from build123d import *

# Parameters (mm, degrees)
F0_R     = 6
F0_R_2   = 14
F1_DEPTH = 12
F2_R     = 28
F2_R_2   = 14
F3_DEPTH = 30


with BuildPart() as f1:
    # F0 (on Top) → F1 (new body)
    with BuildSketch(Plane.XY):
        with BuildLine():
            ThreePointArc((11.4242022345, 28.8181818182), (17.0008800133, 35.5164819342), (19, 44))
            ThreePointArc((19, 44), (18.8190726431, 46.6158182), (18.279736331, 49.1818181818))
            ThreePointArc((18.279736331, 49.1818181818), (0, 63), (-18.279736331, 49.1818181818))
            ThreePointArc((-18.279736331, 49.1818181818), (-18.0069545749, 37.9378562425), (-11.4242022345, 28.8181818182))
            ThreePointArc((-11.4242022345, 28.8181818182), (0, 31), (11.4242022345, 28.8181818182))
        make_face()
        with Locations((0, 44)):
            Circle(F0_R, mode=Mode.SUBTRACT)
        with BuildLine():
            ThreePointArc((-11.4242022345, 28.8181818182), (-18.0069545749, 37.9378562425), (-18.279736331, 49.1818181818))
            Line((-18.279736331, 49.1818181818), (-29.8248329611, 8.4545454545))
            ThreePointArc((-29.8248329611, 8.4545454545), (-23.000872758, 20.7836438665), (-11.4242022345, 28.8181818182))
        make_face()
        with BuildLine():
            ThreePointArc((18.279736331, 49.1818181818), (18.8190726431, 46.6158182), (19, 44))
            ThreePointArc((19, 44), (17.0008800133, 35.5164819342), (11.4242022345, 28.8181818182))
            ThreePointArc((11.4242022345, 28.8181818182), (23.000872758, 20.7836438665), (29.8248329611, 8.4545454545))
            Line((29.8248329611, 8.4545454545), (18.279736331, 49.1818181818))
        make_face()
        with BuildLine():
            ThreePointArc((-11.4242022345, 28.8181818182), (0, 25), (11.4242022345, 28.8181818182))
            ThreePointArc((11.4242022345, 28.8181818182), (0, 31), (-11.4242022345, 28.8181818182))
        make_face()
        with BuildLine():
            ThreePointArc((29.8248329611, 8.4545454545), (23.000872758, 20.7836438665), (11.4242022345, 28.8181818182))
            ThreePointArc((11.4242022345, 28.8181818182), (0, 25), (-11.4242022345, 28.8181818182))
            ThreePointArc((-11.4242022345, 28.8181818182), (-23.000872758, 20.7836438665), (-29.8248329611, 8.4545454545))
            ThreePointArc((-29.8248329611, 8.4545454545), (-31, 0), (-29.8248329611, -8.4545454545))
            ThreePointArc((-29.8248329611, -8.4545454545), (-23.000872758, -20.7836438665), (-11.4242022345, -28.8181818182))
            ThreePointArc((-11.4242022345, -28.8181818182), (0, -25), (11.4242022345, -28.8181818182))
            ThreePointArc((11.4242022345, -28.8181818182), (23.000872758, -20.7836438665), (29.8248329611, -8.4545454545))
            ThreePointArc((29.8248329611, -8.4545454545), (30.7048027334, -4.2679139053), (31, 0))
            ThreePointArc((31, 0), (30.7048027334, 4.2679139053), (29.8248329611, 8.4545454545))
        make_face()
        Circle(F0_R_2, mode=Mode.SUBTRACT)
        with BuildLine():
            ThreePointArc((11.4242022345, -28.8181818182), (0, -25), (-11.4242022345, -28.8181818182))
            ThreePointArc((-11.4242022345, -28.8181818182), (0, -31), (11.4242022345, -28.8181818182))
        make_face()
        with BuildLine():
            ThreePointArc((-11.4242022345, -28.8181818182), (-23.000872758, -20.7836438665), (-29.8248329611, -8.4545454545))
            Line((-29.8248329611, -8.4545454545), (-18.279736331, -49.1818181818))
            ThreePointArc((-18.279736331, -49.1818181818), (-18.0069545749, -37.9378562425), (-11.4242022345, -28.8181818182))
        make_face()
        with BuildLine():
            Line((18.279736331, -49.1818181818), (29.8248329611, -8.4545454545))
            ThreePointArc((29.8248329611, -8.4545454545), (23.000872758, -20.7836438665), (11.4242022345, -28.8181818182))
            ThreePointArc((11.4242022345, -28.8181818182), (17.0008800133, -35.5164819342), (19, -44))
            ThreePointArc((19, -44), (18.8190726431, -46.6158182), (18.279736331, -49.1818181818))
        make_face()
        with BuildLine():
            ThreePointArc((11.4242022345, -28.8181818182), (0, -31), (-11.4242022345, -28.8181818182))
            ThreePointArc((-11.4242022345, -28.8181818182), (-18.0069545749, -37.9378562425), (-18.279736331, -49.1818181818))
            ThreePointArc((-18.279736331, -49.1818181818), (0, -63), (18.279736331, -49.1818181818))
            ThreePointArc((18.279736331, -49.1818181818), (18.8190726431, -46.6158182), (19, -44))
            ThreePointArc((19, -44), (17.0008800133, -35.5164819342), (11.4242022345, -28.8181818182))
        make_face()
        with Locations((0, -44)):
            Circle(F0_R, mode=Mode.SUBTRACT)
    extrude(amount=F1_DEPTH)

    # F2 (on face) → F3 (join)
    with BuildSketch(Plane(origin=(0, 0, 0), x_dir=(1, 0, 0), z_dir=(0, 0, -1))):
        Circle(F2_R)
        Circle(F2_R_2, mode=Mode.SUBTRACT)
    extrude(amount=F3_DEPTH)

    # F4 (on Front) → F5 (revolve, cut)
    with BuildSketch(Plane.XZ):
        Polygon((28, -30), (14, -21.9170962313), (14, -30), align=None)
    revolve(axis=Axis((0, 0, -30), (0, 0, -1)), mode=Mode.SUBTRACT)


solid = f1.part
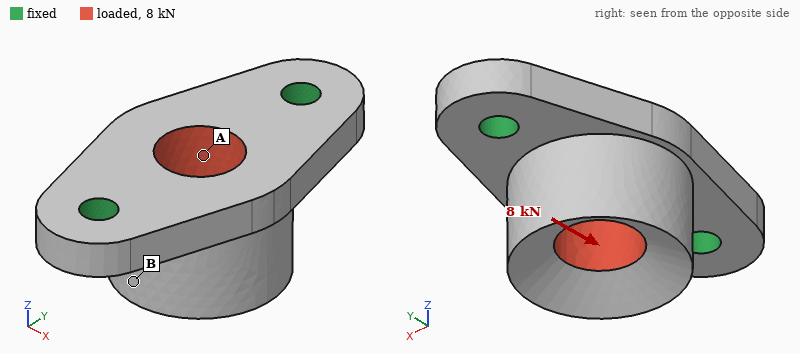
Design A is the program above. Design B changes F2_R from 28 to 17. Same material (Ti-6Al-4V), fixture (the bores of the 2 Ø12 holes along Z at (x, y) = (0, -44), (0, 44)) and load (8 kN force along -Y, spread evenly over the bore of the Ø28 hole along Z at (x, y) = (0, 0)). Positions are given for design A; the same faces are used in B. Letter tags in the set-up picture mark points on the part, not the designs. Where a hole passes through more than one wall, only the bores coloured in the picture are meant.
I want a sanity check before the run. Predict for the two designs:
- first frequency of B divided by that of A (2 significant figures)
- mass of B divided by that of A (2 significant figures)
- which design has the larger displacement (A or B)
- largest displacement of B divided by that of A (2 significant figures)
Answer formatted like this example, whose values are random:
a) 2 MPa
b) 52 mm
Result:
a) 1.6
b) 0.61
c) B
d) 4.3
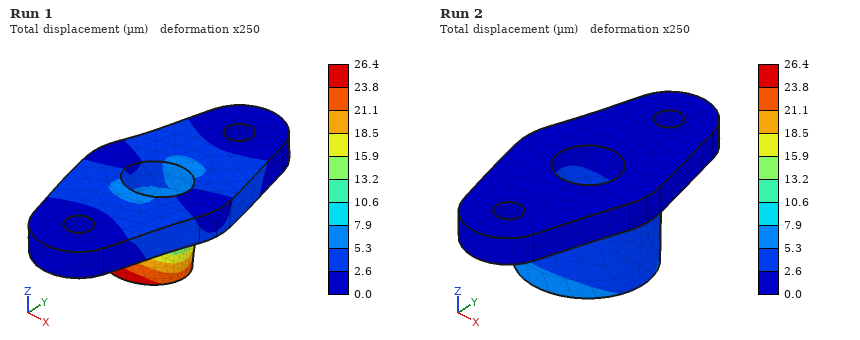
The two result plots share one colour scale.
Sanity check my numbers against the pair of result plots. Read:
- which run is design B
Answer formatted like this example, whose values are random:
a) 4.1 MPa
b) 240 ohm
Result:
a) Run 1
